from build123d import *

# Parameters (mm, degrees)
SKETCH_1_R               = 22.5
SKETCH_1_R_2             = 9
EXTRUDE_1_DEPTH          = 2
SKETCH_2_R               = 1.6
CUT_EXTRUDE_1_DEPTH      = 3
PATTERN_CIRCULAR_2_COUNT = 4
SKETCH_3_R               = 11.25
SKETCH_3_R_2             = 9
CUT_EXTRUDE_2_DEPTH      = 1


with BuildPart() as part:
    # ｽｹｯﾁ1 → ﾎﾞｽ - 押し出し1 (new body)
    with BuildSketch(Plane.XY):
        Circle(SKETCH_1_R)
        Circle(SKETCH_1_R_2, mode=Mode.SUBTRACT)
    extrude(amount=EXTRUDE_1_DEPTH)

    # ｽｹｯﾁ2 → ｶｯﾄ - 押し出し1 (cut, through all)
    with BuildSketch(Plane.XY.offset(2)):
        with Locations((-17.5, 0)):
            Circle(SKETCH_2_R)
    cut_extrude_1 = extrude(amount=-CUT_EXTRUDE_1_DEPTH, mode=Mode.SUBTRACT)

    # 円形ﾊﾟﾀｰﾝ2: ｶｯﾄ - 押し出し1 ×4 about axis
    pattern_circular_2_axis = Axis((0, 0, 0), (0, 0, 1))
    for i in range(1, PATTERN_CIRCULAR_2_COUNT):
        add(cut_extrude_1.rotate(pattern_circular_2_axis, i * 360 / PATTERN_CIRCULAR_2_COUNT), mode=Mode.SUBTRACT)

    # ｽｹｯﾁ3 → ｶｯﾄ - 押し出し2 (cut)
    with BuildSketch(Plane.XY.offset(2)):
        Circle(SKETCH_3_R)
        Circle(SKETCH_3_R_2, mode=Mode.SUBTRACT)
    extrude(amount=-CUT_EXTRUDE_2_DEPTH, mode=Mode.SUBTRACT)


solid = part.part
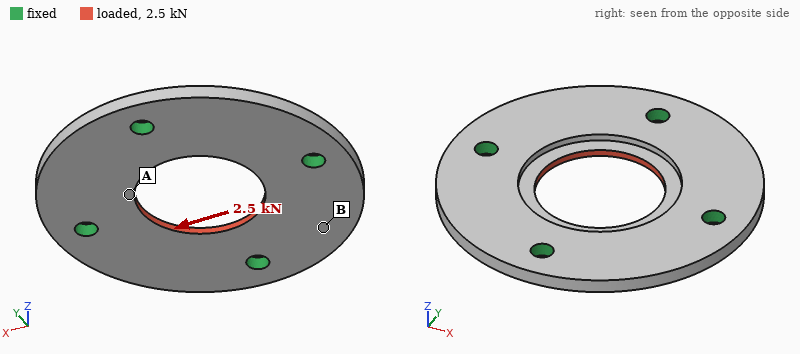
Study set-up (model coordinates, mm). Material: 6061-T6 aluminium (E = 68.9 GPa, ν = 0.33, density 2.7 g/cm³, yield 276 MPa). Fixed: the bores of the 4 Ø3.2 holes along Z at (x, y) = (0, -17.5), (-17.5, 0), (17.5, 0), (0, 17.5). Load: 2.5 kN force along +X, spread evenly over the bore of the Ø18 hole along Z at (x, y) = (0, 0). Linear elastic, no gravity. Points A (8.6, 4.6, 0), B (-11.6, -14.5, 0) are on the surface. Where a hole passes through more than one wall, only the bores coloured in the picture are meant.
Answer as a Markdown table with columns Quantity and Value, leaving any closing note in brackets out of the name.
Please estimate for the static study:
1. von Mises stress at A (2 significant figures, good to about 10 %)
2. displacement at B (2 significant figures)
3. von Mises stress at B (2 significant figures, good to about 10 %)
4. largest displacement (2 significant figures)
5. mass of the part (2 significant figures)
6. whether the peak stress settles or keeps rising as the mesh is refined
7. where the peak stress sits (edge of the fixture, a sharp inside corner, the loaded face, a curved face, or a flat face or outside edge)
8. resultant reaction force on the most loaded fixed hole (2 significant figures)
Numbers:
| Quantity | Value |
|---|---|
| von Mises stress at A | 52 MPa |
| displacement at B | 5.7 µm |
| von Mises stress at B | 12 MPa |
| largest displacement | 12 µm |
| mass of the part | 6.7 g |
| whether the peak stress settles or keeps rising as the mesh is refined | keeps rising |
| where the peak stress sits | edge of the fixture |
| resultant reaction force on the most loaded fixed hole | 670 N |
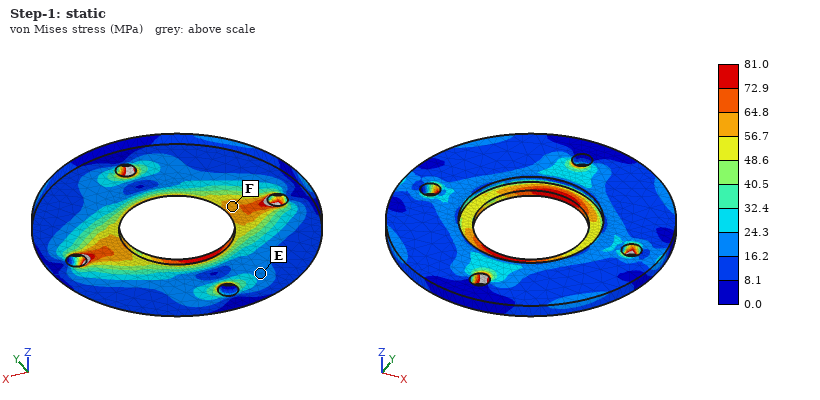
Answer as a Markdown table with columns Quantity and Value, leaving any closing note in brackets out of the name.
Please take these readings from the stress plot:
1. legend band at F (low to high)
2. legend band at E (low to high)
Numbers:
| Quantity | Value |
|---|---|
| legend band at F | 56.7 to 64.8 MPa |
| legend band at E | 16.2 to 24.3 MPa |
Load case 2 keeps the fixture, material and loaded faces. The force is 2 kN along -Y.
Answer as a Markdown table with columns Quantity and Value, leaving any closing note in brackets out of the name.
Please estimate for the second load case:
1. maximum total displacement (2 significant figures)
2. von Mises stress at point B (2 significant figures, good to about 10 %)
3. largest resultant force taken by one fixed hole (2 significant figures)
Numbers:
| Quantity | Value |
|---|---|
| maximum total displacement | 9.9 µm |
| von Mises stress at point B | 9.0 MPa |
| largest resultant force taken by one fixed hole | 540 N |
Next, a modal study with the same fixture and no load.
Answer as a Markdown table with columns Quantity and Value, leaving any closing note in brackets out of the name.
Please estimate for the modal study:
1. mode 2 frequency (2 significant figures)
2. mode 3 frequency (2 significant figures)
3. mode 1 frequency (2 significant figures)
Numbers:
| Quantity | Value |
|---|---|
| mode 2 frequency | 13 kHz |
| mode 3 frequency | 13 kHz |
| mode 1 frequency | 13 kHz |
